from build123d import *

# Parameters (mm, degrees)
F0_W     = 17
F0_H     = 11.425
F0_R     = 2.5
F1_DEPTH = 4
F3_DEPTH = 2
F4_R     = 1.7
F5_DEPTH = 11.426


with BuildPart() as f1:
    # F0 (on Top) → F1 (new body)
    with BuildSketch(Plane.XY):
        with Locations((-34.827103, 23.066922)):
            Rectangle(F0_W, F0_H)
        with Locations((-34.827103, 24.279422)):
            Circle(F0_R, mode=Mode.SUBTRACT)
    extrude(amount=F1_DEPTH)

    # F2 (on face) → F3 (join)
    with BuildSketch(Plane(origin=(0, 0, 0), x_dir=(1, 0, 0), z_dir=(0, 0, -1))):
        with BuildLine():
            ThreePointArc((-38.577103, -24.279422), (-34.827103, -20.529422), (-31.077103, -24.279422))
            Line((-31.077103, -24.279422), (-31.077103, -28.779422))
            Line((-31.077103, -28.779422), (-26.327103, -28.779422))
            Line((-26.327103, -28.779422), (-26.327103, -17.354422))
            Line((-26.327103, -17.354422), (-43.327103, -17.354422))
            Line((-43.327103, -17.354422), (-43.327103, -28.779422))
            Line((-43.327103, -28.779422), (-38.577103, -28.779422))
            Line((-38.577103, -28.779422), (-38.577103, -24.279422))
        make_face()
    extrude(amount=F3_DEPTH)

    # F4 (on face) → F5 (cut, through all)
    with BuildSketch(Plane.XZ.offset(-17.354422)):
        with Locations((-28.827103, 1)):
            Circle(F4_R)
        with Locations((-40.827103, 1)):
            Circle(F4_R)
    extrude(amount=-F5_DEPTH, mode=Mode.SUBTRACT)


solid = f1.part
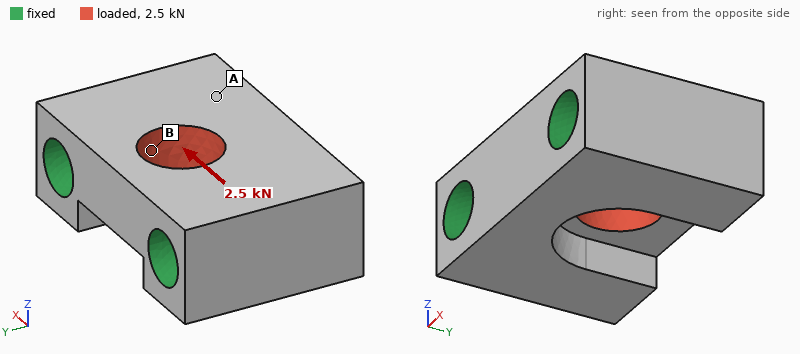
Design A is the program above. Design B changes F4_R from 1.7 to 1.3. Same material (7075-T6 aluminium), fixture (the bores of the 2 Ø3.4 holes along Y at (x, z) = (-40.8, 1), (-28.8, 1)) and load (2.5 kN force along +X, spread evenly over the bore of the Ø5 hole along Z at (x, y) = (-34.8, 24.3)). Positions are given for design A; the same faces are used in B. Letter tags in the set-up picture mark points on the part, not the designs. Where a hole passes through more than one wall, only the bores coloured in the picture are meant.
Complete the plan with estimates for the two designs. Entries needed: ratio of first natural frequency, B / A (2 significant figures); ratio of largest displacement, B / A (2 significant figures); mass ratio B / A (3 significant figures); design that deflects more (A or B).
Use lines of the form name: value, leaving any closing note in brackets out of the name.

ratio of first natural frequency, B / A: 0.87
ratio of largest displacement, B / A: 1.1
mass ratio B / A: 1.11
design that deflects more: B
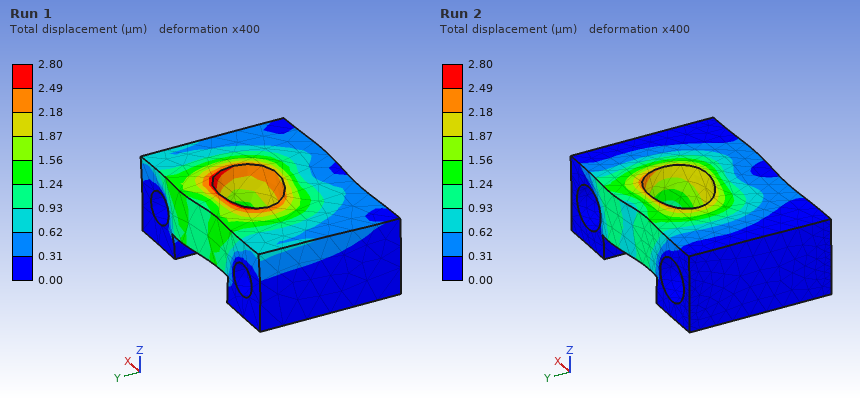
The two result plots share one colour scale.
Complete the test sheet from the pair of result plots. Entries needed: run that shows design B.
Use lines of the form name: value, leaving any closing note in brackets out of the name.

run that shows design B: Run 1
